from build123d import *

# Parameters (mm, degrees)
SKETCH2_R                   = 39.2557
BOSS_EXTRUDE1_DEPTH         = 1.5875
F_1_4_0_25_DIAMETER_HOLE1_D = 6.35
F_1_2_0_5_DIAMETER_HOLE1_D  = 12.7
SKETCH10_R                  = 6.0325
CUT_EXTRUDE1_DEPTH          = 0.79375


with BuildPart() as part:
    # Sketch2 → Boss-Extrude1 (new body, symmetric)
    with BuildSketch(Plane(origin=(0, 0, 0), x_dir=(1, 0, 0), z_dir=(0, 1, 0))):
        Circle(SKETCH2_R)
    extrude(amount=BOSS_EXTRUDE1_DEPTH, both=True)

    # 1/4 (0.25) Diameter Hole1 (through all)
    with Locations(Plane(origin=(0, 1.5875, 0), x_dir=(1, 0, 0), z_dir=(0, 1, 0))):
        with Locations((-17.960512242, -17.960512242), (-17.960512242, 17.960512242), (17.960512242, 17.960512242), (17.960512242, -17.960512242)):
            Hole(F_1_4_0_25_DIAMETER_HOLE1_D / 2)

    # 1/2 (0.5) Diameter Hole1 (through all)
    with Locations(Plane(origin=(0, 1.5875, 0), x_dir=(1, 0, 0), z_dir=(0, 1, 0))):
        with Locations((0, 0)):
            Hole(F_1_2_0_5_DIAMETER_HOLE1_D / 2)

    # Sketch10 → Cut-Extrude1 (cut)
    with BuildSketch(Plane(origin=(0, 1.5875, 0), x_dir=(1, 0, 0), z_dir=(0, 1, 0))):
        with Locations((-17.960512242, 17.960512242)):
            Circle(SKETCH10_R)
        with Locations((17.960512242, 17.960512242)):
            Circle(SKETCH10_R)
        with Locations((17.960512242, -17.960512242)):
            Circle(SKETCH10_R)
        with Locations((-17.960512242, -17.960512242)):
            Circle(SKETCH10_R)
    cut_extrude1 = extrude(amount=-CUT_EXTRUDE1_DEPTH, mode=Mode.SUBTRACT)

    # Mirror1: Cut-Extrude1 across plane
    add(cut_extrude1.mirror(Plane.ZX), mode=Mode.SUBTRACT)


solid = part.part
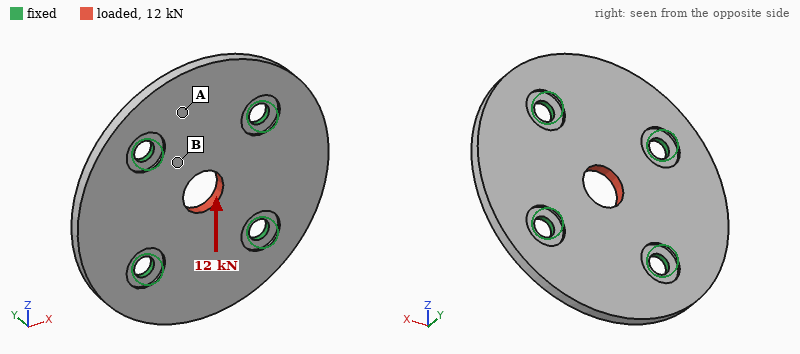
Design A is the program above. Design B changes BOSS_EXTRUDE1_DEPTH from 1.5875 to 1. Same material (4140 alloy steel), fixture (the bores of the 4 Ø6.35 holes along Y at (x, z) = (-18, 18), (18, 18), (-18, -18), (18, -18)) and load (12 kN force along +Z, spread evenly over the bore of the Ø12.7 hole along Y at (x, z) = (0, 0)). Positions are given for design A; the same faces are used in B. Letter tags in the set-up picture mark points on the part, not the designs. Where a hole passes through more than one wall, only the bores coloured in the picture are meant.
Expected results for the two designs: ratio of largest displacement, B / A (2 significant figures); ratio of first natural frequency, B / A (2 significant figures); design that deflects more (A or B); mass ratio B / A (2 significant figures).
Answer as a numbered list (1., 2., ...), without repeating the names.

1. 1.4
2. 0.85
3. B
4. 0.64
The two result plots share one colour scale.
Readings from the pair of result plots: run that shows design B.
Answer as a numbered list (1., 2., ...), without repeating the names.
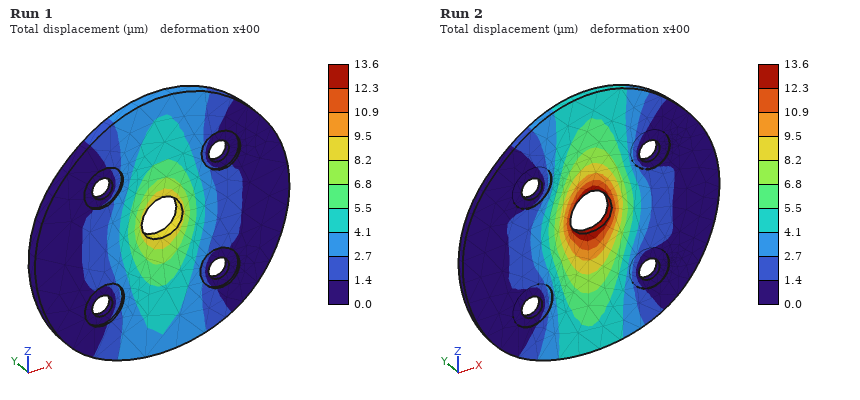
1. Run 2
